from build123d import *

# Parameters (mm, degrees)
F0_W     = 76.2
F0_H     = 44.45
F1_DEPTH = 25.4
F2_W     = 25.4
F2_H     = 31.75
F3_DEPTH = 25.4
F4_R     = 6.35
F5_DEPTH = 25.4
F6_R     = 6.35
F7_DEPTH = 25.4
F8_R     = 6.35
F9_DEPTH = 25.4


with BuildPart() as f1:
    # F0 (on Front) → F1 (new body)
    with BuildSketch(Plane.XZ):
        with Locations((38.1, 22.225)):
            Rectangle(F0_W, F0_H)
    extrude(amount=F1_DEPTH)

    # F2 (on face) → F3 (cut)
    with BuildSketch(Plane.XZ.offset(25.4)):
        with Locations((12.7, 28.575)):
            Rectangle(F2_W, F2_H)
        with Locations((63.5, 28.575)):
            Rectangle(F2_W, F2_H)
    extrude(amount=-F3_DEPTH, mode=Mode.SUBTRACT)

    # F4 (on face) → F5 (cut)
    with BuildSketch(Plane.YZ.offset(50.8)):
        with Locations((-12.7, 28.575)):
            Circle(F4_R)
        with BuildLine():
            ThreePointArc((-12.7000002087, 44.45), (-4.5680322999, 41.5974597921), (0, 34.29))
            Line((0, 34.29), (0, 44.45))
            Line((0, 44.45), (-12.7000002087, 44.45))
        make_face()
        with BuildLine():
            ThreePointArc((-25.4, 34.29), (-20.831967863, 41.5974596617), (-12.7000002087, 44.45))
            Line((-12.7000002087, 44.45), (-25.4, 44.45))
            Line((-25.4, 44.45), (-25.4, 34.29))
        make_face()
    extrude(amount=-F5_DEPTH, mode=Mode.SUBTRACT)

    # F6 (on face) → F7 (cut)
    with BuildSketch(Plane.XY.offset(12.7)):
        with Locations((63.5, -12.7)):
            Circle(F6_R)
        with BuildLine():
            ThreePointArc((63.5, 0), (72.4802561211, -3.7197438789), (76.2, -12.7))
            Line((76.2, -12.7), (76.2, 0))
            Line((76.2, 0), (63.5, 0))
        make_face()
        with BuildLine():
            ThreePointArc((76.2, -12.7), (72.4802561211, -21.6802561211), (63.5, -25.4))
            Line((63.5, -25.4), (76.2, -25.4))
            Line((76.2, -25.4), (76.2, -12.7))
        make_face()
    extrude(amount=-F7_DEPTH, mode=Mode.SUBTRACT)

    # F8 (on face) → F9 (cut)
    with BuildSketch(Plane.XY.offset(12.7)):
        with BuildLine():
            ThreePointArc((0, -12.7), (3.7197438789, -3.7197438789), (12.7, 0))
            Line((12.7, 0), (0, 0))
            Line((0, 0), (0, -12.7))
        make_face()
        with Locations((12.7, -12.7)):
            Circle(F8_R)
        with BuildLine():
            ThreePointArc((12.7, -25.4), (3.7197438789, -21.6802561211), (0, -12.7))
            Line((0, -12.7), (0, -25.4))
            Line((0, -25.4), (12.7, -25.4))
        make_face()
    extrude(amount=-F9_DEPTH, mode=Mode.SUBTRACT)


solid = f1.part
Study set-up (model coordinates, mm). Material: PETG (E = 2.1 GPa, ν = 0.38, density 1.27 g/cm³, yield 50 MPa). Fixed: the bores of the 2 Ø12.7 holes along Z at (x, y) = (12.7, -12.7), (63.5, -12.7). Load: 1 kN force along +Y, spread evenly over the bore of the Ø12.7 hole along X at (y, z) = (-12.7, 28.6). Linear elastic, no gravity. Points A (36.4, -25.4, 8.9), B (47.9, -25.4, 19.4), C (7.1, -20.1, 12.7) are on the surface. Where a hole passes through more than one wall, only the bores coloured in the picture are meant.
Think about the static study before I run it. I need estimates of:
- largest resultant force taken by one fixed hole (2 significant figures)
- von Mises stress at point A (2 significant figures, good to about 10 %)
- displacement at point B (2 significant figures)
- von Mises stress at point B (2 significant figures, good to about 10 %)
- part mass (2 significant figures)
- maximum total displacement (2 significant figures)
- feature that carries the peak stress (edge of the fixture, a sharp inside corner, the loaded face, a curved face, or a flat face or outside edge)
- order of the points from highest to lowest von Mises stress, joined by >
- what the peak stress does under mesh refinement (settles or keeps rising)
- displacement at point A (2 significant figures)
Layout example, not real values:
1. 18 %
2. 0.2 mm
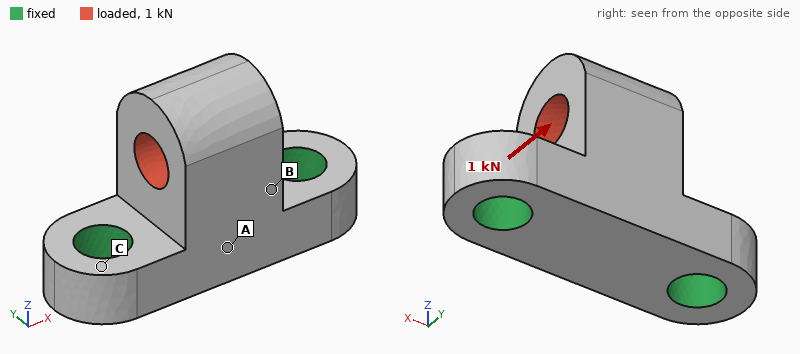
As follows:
1. 500 N
2. 3.5 MPa
3. 0.28 mm
4. 6.4 MPa
5. 45 g
6. 0.64 mm
7. edge of the fixture
8. B > A > C
9. keeps rising
10. 0.18 mm
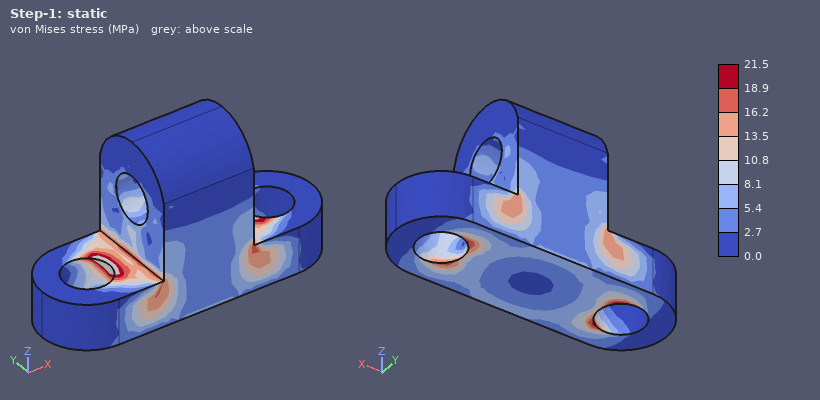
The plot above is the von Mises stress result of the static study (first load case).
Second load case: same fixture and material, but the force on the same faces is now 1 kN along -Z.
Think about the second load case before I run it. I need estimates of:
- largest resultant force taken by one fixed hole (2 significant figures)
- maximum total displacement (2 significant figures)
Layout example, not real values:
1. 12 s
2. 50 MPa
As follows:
1. 530 N
2. 68 µm
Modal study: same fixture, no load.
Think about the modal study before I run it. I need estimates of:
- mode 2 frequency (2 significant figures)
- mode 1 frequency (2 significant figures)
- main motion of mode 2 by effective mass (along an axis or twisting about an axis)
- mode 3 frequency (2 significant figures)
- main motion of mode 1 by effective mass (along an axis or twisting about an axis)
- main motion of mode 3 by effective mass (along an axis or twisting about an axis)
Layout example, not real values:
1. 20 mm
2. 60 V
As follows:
1. 2800 Hz
2. 1700 Hz
3. along X
4. 4200 Hz
5. along Y
6. along Z
